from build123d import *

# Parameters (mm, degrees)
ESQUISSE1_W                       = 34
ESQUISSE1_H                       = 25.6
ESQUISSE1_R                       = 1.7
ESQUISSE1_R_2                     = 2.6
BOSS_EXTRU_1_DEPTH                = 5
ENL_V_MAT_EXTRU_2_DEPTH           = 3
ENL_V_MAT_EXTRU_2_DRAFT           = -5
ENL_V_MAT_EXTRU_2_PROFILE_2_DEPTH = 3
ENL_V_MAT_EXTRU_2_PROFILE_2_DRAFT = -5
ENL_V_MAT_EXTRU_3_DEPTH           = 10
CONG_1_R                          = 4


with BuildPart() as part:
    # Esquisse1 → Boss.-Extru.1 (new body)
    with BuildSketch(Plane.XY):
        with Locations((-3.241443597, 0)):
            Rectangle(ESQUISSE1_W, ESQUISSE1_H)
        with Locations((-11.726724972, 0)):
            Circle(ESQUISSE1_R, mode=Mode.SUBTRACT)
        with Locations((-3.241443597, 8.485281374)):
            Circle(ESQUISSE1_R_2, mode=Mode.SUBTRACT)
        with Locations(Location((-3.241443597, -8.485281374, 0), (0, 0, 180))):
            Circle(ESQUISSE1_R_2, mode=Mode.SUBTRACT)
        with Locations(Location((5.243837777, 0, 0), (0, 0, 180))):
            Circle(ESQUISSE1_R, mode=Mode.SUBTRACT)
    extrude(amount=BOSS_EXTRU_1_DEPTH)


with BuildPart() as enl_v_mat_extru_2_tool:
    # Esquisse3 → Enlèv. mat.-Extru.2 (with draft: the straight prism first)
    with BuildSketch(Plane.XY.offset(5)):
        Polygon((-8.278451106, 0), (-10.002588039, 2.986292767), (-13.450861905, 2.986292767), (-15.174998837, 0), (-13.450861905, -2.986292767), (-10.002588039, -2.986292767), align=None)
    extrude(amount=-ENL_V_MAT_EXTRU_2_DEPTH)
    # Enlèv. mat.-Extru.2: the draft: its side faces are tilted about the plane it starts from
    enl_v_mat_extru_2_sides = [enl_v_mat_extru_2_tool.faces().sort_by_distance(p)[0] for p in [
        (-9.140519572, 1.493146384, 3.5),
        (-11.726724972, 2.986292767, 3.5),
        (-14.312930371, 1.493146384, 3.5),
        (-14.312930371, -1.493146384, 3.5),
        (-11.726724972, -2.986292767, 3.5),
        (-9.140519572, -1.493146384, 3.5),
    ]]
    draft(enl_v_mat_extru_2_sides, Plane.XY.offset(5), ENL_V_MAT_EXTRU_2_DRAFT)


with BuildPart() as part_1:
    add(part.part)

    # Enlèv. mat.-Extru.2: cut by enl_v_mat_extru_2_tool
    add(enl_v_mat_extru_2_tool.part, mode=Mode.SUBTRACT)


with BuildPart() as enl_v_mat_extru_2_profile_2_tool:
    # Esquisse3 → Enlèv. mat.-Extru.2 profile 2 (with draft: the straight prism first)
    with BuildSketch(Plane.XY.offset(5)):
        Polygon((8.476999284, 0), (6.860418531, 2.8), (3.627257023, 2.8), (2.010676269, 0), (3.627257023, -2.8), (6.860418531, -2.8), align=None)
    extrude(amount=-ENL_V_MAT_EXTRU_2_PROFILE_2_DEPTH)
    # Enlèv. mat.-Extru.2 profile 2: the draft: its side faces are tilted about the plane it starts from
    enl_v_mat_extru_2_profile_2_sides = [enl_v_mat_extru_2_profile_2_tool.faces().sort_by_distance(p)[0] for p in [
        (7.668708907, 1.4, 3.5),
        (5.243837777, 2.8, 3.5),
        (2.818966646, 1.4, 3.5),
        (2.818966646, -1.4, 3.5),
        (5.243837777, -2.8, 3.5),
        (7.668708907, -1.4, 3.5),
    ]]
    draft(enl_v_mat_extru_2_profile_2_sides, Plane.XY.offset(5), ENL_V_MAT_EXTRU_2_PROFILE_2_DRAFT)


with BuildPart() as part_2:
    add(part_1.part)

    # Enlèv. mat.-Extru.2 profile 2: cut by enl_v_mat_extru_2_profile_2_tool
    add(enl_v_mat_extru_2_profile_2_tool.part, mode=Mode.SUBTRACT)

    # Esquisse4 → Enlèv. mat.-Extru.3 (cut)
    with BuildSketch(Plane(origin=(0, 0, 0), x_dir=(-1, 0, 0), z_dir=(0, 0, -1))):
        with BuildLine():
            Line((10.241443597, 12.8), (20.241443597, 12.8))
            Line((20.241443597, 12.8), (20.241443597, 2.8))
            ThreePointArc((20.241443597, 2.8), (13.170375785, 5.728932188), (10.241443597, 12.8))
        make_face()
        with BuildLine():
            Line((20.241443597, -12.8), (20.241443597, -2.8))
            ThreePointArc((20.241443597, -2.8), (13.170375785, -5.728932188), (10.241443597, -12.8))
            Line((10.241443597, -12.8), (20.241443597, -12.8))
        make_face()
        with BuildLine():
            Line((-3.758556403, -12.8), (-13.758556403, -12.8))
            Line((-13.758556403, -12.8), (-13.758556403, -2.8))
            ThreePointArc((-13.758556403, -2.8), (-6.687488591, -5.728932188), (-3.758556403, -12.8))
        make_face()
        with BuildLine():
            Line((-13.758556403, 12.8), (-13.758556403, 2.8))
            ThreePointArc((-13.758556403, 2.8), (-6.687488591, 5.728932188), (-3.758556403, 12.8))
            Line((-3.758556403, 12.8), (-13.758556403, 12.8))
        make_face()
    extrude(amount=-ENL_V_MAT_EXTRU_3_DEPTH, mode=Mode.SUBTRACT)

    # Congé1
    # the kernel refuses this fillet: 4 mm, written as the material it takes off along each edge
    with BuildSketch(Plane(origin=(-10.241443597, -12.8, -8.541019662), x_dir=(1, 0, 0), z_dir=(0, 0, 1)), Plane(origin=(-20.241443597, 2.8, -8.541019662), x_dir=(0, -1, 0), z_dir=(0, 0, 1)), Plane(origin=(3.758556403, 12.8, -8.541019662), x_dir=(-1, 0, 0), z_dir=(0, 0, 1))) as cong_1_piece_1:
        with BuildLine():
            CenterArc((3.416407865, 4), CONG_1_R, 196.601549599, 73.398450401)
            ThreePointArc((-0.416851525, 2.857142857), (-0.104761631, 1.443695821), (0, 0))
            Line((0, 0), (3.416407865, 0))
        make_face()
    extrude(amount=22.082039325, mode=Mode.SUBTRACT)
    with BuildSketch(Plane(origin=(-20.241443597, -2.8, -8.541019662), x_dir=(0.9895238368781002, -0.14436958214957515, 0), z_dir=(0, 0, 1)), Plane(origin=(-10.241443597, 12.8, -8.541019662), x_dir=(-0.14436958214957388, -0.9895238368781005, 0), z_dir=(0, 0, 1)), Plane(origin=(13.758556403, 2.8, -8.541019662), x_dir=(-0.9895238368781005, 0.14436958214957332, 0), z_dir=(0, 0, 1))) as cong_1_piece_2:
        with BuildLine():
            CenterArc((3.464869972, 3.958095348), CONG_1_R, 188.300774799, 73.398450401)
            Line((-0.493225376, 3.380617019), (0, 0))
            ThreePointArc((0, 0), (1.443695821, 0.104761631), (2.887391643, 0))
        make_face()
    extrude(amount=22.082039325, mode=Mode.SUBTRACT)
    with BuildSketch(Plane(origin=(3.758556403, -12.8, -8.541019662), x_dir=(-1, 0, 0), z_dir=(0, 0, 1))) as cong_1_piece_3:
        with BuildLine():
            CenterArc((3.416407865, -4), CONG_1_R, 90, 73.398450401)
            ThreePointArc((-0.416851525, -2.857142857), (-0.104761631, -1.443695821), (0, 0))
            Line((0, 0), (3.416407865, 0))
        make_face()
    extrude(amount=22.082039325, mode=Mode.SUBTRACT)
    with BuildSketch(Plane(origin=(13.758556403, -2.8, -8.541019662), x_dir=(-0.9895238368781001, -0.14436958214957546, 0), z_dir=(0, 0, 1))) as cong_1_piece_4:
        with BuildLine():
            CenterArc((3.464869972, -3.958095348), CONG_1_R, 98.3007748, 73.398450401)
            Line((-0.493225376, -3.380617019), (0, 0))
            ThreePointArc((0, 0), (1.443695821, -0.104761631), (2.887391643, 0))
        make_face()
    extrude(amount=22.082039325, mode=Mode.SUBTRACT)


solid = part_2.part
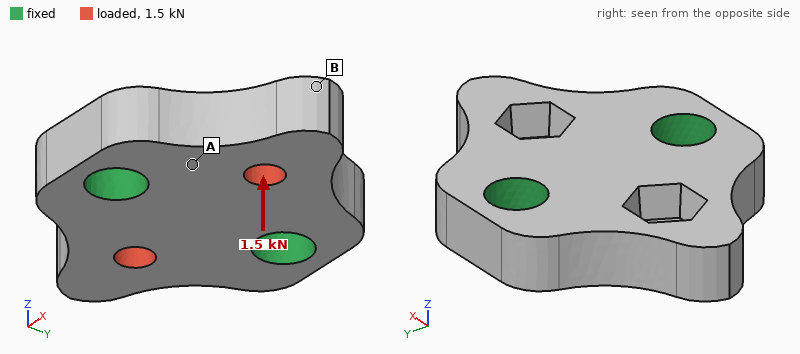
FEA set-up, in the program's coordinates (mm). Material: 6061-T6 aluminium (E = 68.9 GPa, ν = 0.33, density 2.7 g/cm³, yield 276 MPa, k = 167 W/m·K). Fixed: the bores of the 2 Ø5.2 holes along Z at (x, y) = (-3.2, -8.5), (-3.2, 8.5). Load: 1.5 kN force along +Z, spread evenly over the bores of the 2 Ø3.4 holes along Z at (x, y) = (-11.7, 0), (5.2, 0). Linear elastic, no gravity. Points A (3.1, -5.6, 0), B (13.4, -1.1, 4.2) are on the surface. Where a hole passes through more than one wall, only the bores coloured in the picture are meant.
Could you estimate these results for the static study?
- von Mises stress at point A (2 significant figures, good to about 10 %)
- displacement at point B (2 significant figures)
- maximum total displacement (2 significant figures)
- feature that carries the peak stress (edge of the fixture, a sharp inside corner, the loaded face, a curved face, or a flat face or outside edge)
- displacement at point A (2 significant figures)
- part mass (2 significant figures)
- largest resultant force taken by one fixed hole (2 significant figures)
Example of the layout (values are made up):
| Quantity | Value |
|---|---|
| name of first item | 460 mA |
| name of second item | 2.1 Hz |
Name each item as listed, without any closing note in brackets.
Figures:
| Quantity | Value |
|---|---|
| von Mises stress at point A | 37 MPa |
| displacement at point B | 27 µm |
| maximum total displacement | 28 µm |
| feature that carries the peak stress | the loaded face |
| displacement at point A | 6.4 µm |
| part mass | 6.2 g |
| largest resultant force taken by one fixed hole | 750 N |
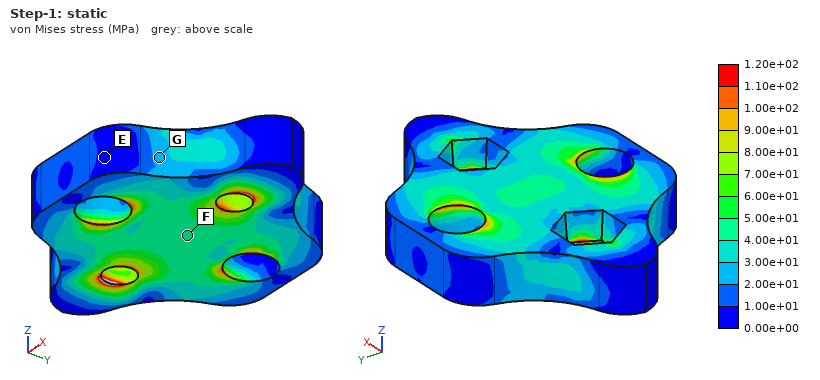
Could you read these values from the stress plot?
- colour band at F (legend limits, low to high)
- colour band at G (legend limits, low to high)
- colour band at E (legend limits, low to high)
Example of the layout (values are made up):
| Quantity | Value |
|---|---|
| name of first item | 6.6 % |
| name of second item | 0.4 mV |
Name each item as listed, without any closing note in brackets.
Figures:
| Quantity | Value |
|---|---|
| colour band at F | 4.00e+01 to 5.00e+01 MPa |
| colour band at G | 2.00e+01 to 3.00e+01 MPa |
| colour band at E | 0.00e+00 to 1.00e+01 MPa |
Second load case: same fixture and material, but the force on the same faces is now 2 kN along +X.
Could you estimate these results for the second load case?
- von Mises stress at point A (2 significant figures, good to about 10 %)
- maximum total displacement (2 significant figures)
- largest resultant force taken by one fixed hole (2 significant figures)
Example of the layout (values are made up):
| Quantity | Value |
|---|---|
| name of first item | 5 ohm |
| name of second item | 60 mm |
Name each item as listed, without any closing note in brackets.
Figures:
| Quantity | Value |
|---|---|
| von Mises stress at point A | 33 MPa |
| maximum total displacement | 16 µm |
| largest resultant force taken by one fixed hole | 1.0 kN |
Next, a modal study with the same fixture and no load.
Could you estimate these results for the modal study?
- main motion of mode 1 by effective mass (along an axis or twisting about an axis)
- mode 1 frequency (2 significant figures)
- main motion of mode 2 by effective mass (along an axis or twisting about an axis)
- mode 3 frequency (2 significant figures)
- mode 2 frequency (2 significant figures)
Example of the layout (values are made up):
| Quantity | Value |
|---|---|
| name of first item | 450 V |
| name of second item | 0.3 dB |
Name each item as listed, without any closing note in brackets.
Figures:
| Quantity | Value |
|---|---|
| main motion of mode 1 by effective mass | twisting about Y |
| mode 1 frequency | 22 kHz |
| main motion of mode 2 by effective mass | along Z |
| mode 3 frequency | 58 kHz |
| mode 2 frequency | 23 kHz |
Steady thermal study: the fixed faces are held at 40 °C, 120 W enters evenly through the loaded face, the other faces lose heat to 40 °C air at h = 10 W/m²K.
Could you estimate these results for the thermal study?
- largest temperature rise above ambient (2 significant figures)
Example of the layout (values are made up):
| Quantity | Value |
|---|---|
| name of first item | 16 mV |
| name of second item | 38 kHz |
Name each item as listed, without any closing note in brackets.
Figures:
| Quantity | Value |
|---|---|
| largest temperature rise above ambient | 70 K |
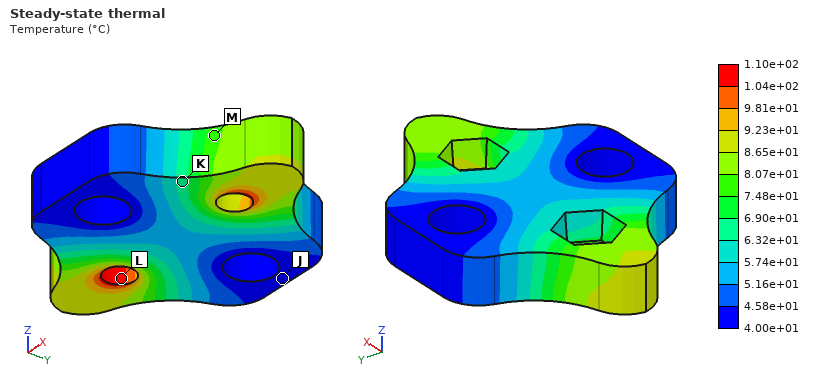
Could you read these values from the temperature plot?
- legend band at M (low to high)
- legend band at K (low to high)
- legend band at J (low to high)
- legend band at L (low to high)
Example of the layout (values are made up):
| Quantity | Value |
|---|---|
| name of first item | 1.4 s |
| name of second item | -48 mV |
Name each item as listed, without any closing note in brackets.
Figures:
| Quantity | Value |
|---|---|
| legend band at M | 7.48e+01 to 8.07e+01 °C |
| legend band at K | 6.32e+01 to 6.90e+01 °C |
| legend band at J | 4.00e+01 to 4.58e+01 °C |
| legend band at L | 1.04e+02 to 1.10e+02 °C |
